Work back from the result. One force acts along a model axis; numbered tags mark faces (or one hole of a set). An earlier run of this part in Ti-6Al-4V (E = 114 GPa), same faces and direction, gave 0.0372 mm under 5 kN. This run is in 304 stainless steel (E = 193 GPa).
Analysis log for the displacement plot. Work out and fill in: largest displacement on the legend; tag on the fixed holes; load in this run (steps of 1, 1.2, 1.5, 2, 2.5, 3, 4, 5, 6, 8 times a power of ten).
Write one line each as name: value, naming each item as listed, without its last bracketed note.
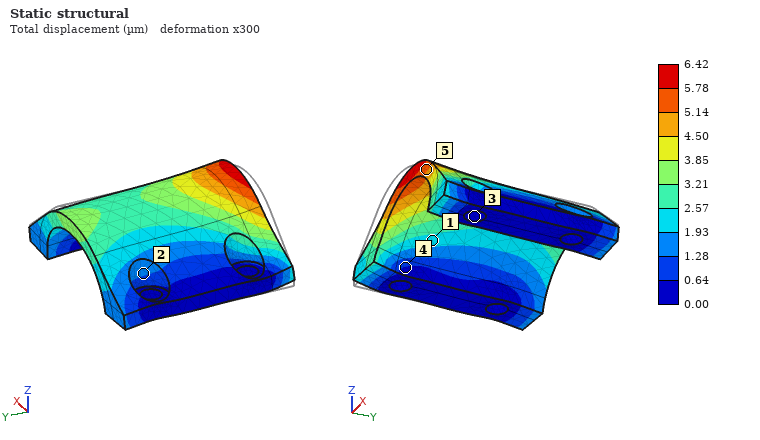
largest displacement on the legend: 6.42 µm
tag on the fixed holes: 3
load in this run: 1.5 kN
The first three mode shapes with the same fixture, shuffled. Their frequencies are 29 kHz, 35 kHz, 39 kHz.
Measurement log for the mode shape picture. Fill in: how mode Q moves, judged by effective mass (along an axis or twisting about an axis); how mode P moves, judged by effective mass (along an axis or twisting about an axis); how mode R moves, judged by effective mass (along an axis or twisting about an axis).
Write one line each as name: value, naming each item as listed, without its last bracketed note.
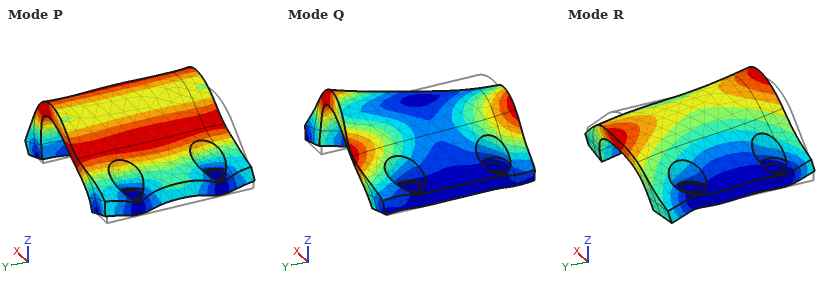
how mode Q moves, judged by effective mass: twisting about Z
how mode P moves, judged by effective mass: along X
how mode R moves, judged by effective mass: along Y
